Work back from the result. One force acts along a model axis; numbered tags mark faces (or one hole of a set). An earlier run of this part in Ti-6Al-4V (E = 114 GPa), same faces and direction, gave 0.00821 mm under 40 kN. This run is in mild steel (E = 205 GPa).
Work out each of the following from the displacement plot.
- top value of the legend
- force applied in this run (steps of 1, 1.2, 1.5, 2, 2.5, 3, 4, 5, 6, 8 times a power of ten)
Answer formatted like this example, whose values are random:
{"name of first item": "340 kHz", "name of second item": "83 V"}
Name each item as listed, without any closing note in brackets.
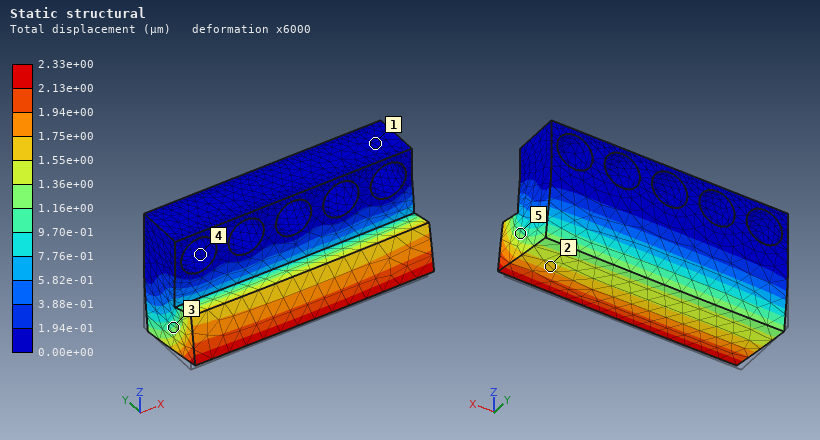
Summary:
{"top value of the legend": "2.33e+00 µm", "force applied in this run": "20 kN"}
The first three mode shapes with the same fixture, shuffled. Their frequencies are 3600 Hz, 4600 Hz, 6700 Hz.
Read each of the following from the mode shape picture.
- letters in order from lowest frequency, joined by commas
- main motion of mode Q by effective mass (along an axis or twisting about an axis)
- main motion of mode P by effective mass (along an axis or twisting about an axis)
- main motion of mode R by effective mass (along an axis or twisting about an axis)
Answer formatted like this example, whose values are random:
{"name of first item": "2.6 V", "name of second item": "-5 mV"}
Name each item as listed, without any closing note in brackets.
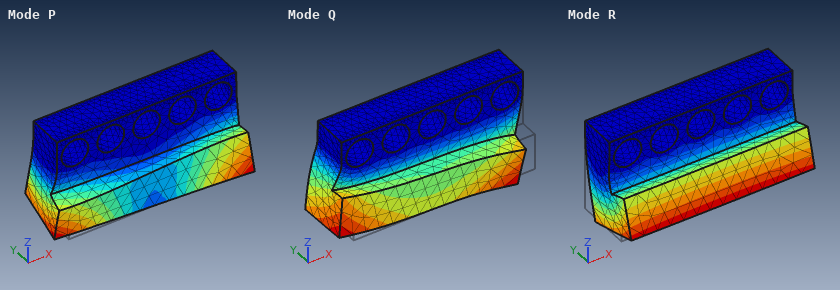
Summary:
{"letters in order from lowest frequency, joined by commas": "R, P, Q", "main motion of mode Q by effective mass": "along X", "main motion of mode P by effective mass": "twisting about Z", "main motion of mode R by effective mass": "along Y"}
